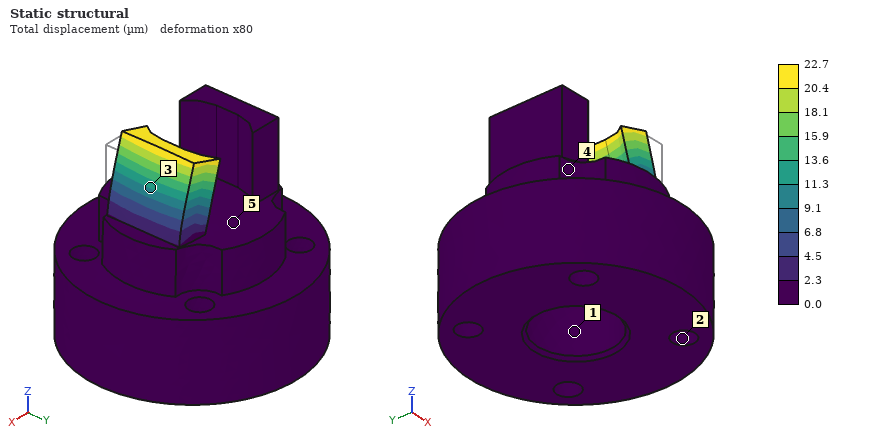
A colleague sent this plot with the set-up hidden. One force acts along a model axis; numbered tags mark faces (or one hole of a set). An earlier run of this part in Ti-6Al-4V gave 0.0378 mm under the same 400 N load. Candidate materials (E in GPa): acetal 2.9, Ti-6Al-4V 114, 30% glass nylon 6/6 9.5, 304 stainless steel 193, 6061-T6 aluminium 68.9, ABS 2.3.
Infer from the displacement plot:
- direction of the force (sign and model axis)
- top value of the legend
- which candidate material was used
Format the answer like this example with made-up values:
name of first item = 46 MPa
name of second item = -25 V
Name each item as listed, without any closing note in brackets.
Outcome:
direction of the force = -X
top value of the legend = 22.7 µm
which candidate material was used = 304 stainless steel
